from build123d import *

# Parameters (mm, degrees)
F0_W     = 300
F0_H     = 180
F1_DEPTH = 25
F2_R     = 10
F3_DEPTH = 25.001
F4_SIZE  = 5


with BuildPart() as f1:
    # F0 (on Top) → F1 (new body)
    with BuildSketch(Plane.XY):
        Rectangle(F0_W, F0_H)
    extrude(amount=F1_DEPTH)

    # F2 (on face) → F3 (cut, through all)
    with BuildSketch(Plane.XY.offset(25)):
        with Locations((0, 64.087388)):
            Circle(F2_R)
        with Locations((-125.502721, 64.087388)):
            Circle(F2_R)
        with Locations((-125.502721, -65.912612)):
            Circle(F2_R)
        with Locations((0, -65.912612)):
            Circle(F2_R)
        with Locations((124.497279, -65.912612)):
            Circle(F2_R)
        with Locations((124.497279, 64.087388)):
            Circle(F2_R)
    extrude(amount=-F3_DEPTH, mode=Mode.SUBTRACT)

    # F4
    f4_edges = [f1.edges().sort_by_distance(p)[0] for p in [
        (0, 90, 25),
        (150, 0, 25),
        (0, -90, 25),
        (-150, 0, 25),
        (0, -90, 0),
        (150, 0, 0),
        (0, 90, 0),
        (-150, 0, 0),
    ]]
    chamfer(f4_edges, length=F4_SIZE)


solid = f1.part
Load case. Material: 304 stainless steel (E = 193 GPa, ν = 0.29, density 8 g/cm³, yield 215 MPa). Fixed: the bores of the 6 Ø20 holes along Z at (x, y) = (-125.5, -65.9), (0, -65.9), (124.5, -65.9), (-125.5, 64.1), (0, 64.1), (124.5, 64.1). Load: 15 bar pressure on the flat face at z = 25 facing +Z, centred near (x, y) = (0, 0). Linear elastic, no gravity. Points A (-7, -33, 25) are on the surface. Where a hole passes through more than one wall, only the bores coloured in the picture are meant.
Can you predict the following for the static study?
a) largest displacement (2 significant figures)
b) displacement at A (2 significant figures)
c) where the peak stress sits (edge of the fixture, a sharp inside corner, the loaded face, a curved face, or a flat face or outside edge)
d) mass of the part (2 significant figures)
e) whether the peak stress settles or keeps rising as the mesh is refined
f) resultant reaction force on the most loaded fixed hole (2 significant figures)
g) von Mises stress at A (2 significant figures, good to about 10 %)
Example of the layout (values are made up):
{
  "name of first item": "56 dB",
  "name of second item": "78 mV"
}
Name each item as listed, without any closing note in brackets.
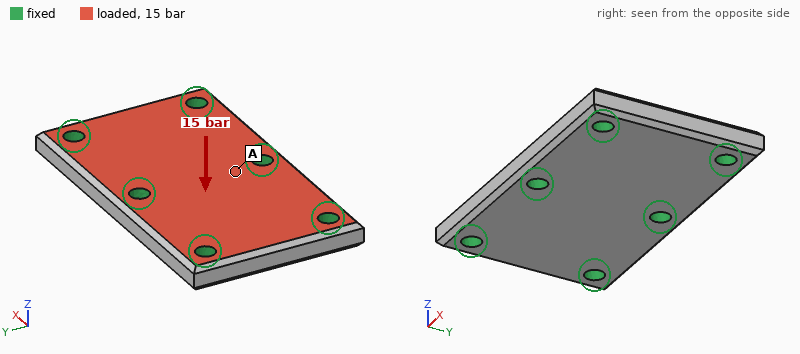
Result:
{
  "largest displacement": "10 µm",
  "displacement at A": "5.7 µm",
  "where the peak stress sits": "edge of the fixture",
  "mass of the part": "10 kg",
  "whether the peak stress settles or keeps rising as the mesh is refined": "keeps rising",
  "resultant reaction force on the most loaded fixed hole": "16 kN",
  "von Mises stress at A": "9.0 MPa"
}
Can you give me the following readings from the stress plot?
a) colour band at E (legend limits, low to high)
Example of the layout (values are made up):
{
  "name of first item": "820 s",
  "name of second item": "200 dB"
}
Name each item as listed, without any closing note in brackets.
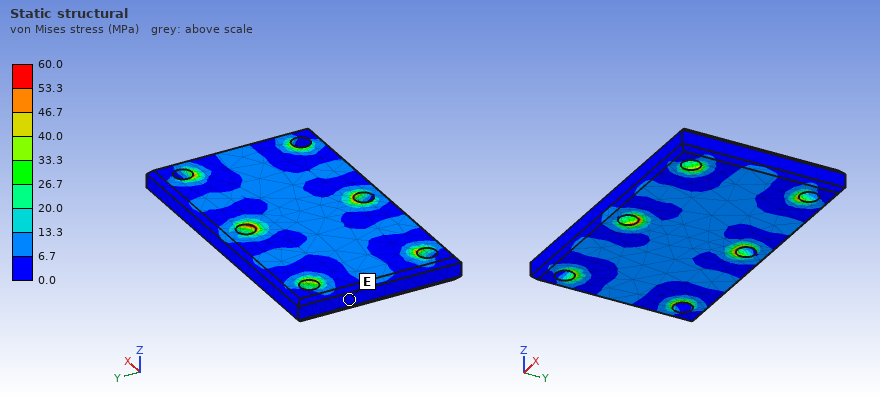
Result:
{
  "colour band at E": "0.0 to 6.7 MPa"
}
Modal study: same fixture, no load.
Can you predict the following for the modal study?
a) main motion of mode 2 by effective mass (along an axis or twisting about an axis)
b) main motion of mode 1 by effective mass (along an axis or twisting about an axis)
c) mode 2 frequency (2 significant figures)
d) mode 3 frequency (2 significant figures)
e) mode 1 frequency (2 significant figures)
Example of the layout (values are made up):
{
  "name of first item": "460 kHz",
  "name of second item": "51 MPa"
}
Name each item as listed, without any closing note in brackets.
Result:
{
  "main motion of mode 2 by effective mass": "twisting about Y",
  "main motion of mode 1 by effective mass": "along Z",
  "mode 2 frequency": "5300 Hz",
  "mode 3 frequency": "7500 Hz",
  "mode 1 frequency": "5000 Hz"
}
